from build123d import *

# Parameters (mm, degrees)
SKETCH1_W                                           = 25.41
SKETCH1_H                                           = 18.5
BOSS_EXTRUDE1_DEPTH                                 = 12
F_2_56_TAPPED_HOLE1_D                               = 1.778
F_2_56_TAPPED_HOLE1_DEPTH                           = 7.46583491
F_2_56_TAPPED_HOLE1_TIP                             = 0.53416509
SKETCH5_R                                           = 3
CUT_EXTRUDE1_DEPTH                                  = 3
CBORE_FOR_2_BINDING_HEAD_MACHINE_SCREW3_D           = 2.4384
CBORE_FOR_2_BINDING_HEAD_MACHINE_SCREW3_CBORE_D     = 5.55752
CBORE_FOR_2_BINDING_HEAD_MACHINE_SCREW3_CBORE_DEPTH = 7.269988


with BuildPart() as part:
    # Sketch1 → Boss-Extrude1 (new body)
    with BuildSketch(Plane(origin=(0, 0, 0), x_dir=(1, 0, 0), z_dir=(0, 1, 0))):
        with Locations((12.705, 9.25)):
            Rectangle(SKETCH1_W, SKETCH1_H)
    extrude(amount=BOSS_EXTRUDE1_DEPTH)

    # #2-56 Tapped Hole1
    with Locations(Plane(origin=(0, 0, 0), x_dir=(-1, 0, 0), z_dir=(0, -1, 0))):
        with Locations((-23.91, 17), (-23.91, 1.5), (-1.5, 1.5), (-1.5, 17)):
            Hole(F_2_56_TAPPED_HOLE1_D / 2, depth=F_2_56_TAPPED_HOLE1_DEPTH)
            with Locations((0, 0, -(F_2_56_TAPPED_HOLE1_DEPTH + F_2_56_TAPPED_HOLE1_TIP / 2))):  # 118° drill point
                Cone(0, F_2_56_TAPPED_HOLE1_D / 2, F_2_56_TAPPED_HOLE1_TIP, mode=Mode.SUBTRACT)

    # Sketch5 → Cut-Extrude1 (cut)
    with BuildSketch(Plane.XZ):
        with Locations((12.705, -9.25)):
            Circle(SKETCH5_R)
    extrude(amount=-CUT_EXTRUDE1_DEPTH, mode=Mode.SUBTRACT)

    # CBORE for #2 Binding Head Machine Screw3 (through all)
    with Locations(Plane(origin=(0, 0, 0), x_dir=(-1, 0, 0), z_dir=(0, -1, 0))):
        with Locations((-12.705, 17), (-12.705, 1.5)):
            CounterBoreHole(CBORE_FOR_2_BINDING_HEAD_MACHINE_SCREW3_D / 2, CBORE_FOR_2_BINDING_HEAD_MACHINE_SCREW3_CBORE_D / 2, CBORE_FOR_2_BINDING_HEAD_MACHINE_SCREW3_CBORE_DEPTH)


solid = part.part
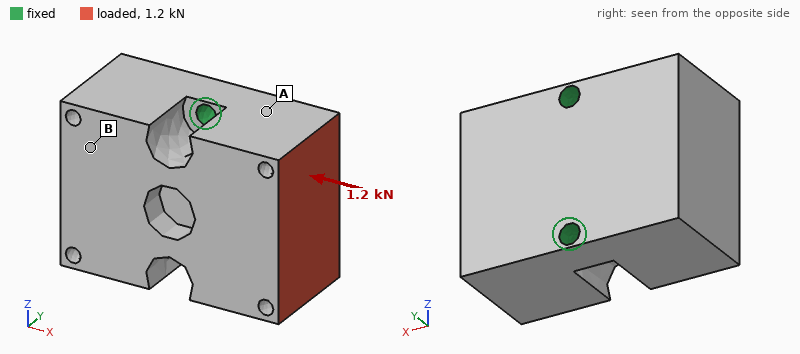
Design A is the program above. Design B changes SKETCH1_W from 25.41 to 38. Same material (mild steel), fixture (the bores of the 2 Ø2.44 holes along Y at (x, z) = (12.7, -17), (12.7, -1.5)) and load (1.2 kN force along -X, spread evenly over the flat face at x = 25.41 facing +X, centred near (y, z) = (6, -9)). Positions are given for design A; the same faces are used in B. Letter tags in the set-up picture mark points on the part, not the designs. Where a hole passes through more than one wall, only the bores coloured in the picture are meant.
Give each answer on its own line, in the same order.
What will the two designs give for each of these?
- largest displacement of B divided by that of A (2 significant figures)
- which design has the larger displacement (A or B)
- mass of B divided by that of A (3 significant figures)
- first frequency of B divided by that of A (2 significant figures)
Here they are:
1.3
B
1.54
0.58
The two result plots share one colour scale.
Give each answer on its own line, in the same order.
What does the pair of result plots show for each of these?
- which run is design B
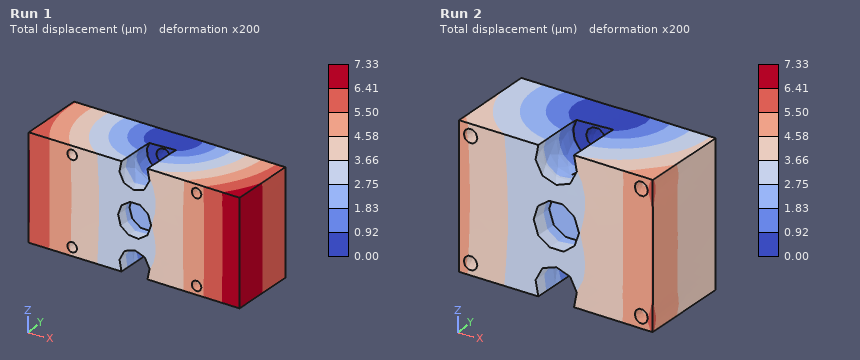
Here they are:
Run 1
